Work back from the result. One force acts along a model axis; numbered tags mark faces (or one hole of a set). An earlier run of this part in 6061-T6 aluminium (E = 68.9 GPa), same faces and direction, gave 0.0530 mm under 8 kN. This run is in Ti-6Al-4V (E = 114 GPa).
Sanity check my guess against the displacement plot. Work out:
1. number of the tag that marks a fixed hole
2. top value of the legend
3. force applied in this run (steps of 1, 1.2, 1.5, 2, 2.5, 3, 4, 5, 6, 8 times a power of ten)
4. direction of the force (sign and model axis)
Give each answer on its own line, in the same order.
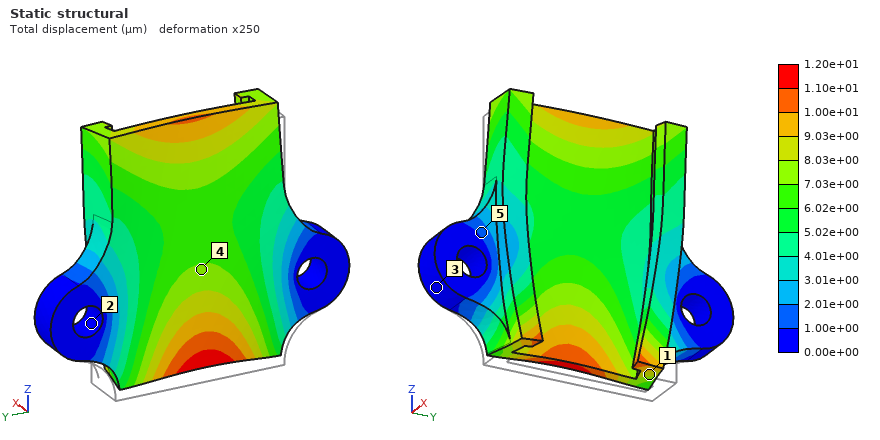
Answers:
2
1.20e+01 µm
3 kN
+Z
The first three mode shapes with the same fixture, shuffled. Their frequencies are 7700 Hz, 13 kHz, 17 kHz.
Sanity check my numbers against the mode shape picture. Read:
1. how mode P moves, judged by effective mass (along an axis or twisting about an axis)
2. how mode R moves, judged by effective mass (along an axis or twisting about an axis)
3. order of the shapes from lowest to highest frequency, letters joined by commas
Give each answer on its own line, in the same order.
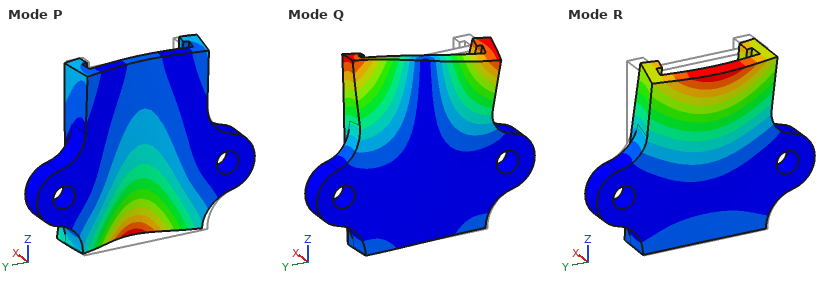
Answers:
along X
along X
R, Q, P
